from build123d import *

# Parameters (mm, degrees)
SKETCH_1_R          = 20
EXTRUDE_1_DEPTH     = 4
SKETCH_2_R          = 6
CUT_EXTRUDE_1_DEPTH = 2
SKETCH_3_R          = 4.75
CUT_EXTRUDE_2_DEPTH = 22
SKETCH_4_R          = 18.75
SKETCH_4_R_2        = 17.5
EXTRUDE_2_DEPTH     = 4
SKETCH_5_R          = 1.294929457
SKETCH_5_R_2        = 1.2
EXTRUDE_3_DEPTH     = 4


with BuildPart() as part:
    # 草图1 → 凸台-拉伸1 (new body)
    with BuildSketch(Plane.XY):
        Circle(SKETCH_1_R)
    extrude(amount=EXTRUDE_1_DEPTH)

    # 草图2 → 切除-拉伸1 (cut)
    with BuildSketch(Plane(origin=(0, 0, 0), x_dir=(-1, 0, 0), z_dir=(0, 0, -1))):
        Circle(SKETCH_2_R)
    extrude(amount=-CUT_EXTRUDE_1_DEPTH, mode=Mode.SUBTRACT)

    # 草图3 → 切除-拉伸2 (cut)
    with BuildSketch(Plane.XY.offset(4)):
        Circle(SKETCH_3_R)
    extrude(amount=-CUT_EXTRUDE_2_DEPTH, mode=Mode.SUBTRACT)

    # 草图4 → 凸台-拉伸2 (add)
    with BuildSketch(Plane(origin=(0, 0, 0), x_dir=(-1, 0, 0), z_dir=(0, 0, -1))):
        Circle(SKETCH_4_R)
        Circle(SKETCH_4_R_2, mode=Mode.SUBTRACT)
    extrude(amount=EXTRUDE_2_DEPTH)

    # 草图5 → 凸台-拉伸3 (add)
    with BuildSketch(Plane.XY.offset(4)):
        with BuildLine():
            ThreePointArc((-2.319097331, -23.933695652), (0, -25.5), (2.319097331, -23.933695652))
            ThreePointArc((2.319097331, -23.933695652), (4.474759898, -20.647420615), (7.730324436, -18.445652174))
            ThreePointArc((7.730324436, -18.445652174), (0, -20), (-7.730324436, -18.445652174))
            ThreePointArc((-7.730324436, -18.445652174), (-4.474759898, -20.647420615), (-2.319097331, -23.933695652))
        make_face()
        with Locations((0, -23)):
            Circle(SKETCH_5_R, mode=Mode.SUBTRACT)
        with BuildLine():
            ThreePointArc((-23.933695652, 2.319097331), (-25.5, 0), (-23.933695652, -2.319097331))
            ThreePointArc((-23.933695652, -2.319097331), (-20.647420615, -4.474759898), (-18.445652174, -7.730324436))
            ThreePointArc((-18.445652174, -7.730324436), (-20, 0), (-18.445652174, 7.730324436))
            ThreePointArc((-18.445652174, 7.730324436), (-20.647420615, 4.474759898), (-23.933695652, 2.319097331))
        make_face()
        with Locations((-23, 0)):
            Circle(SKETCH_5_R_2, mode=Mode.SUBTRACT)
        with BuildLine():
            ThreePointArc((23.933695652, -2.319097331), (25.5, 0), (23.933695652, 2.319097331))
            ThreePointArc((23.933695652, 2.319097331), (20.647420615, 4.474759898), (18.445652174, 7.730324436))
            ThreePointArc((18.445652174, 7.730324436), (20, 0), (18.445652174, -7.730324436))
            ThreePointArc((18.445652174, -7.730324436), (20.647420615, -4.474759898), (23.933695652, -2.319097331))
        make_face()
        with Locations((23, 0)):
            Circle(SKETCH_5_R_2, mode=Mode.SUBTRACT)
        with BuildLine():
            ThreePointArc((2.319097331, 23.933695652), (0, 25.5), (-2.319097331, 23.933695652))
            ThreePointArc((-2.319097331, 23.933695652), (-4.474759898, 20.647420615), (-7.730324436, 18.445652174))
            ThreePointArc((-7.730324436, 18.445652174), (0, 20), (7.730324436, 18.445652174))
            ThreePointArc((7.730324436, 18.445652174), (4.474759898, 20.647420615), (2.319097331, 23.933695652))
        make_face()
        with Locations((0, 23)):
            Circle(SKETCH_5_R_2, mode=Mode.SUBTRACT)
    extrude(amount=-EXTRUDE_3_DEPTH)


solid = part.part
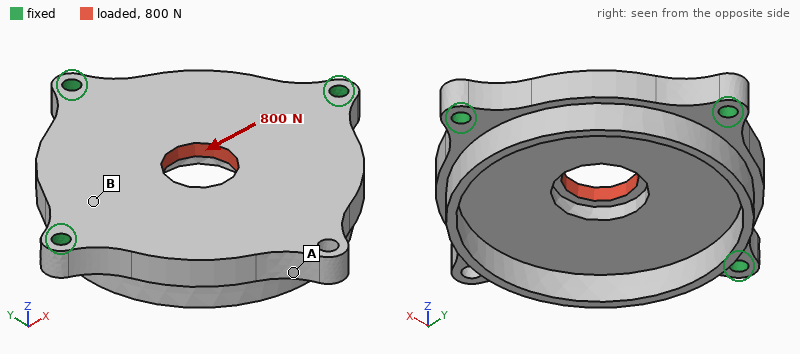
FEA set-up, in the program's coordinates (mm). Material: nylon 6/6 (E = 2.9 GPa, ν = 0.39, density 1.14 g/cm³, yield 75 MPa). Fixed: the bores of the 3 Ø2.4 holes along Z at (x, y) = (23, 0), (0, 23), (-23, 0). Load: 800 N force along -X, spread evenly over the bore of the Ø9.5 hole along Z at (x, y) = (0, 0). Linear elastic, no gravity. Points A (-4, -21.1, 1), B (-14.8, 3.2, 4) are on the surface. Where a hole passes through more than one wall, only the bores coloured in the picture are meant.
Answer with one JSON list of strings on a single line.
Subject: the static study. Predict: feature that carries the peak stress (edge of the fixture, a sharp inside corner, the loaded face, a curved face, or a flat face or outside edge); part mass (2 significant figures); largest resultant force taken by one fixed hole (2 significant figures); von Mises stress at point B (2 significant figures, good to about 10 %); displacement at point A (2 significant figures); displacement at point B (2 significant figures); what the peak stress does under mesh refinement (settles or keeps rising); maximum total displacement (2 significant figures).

["edge of the fixture", "6.5 g", "360 N", "8.8 MPa", "40 µm", "34 µm", "keeps rising", "75 µm"]
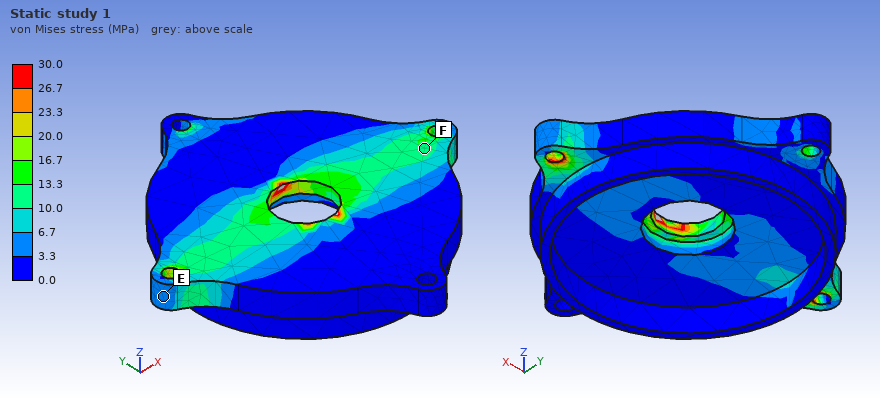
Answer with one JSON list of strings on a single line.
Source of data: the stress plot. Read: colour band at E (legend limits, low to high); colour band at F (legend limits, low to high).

["3.3 to 6.7 MPa", "10.0 to 13.3 MPa"]
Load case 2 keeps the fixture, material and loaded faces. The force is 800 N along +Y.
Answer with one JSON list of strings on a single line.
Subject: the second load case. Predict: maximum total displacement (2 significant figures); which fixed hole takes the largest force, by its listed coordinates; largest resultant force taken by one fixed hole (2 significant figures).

["0.29 mm", "(0, 23)", "420 N"]
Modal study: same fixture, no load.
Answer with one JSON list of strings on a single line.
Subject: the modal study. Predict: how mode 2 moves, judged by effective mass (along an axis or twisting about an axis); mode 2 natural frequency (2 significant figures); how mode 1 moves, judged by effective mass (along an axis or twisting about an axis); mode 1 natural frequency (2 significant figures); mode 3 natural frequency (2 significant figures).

["along Z", "4300 Hz", "along Z", "1500 Hz", "4900 Hz"]
